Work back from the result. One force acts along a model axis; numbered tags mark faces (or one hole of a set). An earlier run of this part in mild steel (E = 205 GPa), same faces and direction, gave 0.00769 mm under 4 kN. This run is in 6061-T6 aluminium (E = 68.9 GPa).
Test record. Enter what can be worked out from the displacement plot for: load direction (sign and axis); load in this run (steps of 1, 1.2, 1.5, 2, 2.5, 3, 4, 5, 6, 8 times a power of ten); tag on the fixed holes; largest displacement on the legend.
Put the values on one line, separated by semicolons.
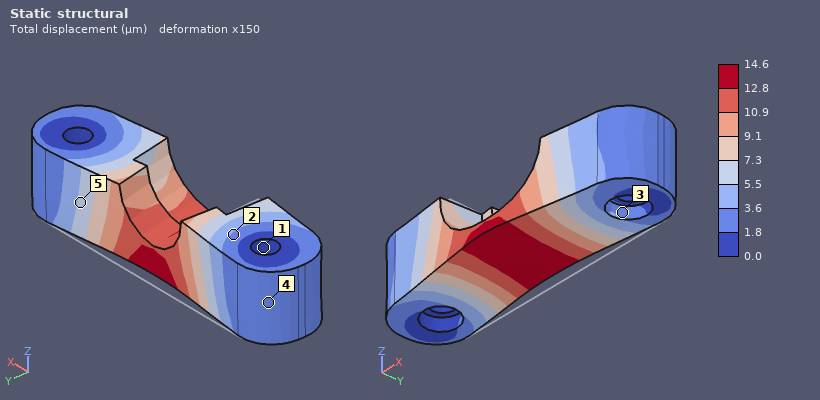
-Y; 2.5 kN; 1; 14.6 µm
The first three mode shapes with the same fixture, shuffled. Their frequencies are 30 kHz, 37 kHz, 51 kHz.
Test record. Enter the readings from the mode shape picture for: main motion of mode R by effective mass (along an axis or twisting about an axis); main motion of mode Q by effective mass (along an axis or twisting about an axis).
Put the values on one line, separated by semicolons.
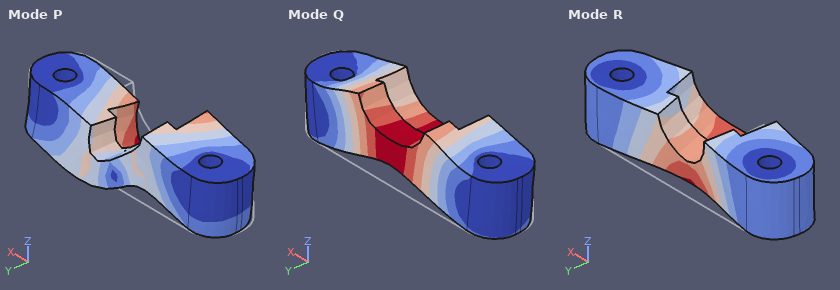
along Y; along Z
